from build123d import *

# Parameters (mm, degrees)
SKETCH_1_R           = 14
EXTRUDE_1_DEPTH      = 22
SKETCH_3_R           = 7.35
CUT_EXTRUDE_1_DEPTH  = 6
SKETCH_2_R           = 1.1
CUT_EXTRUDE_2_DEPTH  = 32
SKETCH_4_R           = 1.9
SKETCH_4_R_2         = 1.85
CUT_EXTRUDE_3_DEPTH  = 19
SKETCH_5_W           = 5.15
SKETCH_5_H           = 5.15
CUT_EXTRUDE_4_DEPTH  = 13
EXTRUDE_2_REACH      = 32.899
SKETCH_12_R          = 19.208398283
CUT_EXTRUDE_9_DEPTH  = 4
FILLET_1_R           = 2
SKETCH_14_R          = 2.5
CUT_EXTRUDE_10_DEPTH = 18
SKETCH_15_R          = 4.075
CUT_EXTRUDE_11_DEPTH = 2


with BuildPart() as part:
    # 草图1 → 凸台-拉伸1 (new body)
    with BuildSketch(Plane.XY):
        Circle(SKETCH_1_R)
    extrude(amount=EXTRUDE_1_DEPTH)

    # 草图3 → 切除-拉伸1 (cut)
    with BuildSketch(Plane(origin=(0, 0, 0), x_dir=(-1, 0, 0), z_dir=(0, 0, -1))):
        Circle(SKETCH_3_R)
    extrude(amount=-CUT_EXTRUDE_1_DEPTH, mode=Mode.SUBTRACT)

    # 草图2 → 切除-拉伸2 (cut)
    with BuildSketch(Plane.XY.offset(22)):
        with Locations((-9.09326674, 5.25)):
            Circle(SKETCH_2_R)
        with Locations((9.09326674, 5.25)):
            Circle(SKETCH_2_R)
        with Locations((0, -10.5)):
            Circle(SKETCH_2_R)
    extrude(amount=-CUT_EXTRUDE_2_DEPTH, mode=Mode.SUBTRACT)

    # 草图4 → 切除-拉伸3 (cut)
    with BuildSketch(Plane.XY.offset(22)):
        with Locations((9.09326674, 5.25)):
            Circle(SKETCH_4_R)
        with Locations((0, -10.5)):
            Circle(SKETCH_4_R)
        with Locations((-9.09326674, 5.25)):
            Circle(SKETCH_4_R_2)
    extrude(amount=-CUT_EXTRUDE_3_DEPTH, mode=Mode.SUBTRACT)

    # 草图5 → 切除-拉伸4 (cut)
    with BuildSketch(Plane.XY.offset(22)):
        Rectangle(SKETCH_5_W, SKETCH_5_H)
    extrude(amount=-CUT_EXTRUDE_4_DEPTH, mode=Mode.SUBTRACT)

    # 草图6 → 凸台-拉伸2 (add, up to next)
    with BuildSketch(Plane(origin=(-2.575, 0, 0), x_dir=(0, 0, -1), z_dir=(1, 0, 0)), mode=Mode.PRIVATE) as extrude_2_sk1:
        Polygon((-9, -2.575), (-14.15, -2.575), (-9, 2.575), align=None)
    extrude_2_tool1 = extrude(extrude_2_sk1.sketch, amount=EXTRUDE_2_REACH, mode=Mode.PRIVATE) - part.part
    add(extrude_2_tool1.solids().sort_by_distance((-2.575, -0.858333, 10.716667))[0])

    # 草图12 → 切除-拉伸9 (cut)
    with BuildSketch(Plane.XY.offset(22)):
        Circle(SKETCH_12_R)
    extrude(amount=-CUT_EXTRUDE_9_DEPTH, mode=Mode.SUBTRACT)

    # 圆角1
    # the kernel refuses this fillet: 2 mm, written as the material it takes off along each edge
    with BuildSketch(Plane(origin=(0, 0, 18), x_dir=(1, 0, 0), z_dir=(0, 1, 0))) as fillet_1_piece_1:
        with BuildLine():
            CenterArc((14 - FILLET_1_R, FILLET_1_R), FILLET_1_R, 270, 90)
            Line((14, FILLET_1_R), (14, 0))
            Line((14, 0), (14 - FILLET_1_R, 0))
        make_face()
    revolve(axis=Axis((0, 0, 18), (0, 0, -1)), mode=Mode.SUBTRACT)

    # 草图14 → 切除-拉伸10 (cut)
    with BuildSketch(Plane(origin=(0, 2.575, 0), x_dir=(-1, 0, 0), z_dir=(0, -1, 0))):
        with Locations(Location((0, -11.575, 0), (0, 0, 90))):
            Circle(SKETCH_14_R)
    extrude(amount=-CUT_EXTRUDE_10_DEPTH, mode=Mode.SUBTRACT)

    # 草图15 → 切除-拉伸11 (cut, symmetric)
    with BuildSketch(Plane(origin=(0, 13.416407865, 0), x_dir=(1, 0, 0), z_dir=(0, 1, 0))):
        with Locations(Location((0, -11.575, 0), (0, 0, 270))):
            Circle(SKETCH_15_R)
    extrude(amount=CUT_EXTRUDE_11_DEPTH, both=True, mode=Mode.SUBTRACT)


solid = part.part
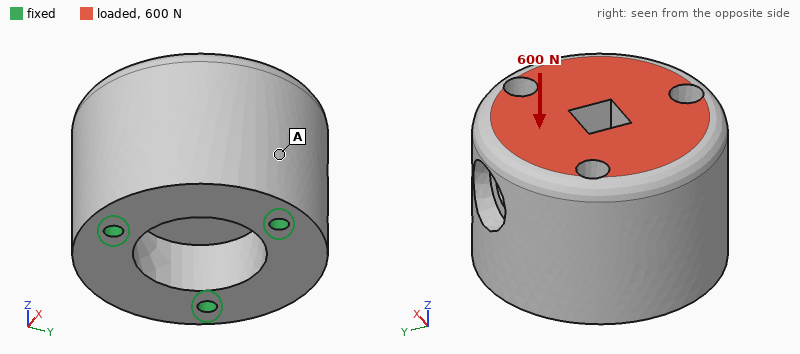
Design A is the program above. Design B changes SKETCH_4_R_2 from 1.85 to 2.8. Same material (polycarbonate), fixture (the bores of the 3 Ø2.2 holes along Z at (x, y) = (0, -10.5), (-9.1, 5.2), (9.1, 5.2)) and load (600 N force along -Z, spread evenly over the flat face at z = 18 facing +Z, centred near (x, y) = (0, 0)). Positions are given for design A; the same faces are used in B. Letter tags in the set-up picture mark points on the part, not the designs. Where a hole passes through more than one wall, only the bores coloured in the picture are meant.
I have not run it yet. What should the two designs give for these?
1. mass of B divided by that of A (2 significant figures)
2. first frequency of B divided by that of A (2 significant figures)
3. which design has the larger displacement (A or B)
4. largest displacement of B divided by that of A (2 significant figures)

0.98
0.94
B
1.1
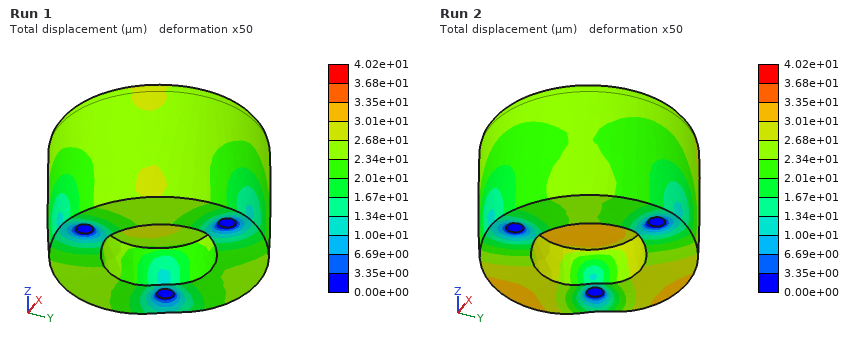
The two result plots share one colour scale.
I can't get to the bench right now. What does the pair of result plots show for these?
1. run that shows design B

Run 2
